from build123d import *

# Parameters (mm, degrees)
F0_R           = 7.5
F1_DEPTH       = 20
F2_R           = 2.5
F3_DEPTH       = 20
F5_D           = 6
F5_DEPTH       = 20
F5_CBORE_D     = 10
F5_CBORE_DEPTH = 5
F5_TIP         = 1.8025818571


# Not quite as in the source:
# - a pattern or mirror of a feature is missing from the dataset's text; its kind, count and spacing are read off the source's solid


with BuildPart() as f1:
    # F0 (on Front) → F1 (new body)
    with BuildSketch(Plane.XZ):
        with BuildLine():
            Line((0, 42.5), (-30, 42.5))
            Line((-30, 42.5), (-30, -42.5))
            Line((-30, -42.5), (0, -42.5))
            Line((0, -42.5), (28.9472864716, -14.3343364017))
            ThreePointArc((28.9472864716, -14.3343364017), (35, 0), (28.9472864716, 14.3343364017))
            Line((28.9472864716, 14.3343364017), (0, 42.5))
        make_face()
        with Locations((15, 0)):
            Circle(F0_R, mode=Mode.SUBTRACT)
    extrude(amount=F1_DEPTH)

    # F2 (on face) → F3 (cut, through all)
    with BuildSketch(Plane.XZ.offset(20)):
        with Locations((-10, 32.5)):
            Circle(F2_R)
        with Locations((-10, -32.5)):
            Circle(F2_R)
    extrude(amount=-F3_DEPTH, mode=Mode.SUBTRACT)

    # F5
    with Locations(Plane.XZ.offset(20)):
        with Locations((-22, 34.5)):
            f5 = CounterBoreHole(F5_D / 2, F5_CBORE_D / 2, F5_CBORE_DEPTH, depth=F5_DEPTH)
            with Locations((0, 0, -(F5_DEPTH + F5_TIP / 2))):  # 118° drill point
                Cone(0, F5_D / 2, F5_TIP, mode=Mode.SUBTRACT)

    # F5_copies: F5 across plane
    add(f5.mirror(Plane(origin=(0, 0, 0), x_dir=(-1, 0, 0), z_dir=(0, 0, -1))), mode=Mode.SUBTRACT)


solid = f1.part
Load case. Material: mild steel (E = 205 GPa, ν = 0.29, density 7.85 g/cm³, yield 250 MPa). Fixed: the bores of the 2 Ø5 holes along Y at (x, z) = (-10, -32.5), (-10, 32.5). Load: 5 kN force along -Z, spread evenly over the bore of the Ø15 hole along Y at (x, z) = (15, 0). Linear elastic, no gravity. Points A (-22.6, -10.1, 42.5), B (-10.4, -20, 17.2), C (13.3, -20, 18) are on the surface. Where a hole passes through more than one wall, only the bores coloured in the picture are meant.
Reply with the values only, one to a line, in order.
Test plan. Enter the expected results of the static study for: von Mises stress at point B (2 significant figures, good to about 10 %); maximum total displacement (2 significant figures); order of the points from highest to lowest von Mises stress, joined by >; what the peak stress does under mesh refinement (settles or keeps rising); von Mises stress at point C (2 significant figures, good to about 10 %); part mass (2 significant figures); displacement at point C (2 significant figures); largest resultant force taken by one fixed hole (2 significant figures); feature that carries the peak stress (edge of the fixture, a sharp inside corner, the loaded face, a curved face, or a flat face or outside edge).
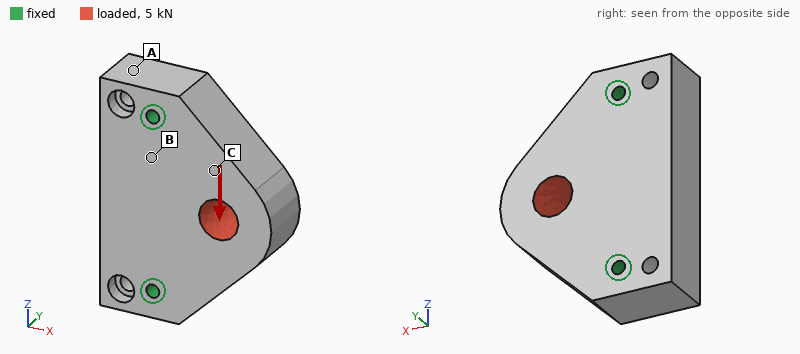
3.7 MPa
2.4 µm
C > B > A
keeps rising
6.8 MPa
630 g
1.4 µm
3.1 kN
edge of the fixture
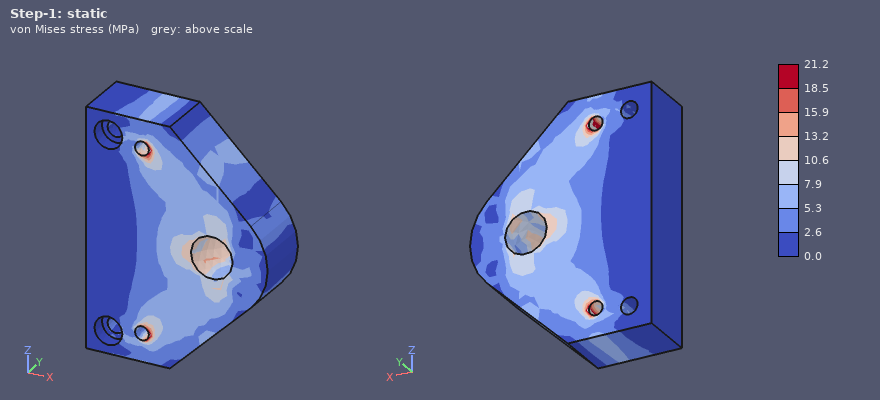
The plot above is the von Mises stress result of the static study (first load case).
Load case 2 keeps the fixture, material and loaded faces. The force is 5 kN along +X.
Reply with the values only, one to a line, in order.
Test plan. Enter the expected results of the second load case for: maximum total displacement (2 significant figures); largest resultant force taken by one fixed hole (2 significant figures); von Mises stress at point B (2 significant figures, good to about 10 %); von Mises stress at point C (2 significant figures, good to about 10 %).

1.8 µm
2.6 kN
4.0 MPa
4.8 MPa
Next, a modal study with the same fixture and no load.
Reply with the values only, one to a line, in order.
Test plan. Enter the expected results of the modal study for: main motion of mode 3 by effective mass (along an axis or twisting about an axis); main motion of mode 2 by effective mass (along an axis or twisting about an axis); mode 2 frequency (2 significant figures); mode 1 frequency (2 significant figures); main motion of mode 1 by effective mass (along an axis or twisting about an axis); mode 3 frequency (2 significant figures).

along X
along Y
13 kHz
6900 Hz
along Y
16 kHz
